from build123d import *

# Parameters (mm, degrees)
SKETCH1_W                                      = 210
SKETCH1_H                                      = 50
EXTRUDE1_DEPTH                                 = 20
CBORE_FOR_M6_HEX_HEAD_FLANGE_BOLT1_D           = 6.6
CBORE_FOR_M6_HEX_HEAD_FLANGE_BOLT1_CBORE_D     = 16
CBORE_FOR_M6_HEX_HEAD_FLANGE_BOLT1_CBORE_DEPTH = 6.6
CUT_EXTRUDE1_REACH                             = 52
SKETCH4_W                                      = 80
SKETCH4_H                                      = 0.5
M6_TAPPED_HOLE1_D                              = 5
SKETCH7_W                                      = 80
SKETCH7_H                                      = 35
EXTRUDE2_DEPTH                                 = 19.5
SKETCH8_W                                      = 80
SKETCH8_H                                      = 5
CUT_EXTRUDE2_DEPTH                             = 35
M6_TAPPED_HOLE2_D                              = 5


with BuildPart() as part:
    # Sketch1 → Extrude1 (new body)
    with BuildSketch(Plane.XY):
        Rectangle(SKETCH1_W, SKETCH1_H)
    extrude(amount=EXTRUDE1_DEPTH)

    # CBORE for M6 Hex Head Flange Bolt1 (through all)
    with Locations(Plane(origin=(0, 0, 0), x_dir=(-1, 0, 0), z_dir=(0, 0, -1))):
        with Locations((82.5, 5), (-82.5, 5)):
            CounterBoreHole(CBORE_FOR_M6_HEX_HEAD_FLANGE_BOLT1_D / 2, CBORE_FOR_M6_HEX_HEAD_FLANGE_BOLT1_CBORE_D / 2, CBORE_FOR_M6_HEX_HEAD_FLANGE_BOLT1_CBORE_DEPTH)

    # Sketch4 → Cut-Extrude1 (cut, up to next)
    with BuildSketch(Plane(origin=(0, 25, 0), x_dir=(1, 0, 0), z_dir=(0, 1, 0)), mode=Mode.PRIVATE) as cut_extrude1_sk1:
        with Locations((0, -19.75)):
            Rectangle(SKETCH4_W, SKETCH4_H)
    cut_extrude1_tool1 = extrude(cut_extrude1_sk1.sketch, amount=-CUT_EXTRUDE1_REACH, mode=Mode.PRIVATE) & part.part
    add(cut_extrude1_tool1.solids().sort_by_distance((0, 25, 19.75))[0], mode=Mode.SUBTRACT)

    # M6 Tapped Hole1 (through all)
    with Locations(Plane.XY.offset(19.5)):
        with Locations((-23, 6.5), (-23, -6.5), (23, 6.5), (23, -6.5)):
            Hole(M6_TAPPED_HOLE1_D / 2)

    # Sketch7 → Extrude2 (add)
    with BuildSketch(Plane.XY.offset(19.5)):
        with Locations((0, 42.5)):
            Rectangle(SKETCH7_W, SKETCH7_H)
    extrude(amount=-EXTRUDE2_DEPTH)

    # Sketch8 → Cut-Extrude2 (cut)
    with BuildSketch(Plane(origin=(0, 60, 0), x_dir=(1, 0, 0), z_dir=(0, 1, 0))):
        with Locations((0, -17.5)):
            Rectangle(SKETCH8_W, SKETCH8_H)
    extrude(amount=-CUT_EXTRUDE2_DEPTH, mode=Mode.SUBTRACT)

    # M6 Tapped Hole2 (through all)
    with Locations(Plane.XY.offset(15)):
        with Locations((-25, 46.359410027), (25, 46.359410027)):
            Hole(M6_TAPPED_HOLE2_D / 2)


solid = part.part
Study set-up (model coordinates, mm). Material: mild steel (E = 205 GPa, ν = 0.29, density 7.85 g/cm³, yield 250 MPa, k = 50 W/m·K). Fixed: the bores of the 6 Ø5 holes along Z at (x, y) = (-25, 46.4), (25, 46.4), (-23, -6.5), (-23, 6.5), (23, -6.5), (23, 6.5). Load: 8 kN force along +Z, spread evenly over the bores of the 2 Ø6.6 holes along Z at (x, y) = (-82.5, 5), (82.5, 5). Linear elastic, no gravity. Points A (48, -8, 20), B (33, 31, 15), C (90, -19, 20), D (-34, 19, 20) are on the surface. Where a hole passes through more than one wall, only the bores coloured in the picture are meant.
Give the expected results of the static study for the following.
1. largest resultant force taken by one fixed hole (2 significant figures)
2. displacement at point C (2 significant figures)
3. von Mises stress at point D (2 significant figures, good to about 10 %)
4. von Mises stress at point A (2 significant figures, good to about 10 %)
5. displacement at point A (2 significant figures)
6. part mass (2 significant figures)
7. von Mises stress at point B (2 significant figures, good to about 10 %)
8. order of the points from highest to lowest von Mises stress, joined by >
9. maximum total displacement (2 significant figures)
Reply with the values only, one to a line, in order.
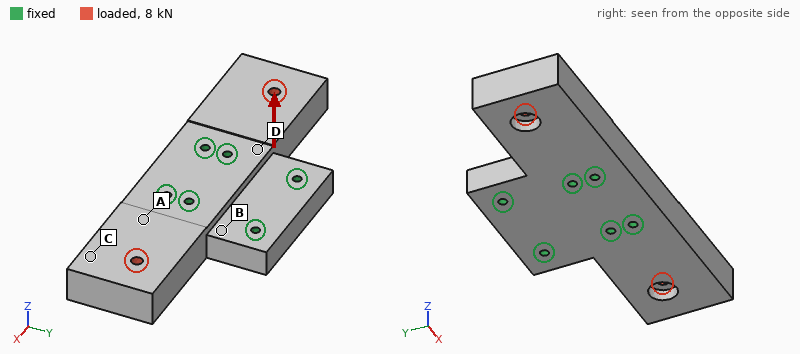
2.6 kN
56 µm
54 MPa
38 MPa
15 µm
1.9 kg
26 MPa
D > A > B > C
79 µm
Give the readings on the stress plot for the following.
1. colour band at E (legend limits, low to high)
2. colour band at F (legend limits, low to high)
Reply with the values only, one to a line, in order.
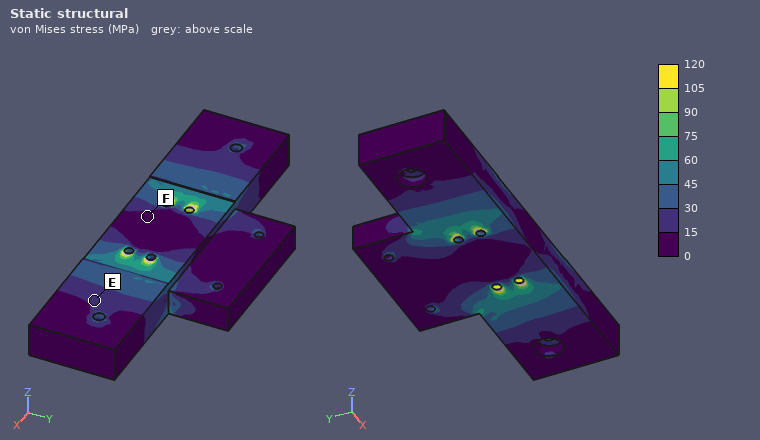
15 to 30 MPa
0 to 15 MPa
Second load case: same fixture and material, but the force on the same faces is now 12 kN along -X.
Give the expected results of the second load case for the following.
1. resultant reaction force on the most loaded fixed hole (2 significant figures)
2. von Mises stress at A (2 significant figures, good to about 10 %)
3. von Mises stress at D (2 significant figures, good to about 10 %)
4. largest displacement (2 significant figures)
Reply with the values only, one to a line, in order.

3.0 kN
11 MPa
12 MPa
11 µm
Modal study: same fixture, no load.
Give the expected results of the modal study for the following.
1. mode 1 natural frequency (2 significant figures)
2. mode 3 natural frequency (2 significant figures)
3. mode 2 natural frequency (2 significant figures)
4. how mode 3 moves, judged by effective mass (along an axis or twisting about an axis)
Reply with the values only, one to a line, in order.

2300 Hz
4600 Hz
2300 Hz
twisting about Z
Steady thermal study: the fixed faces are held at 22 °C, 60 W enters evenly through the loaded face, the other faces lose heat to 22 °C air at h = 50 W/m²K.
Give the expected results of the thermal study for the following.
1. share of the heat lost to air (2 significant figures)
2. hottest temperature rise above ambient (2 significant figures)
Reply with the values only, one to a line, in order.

36 %
35 K
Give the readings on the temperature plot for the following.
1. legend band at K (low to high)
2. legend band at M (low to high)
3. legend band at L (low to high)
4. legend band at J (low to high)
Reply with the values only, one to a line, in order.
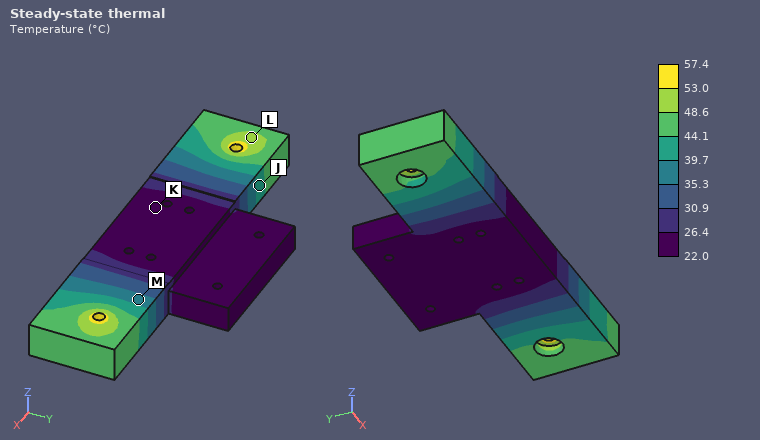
22.0 to 26.4 °C
35.3 to 39.7 °C
48.6 to 53.0 °C
39.7 to 44.1 °C
